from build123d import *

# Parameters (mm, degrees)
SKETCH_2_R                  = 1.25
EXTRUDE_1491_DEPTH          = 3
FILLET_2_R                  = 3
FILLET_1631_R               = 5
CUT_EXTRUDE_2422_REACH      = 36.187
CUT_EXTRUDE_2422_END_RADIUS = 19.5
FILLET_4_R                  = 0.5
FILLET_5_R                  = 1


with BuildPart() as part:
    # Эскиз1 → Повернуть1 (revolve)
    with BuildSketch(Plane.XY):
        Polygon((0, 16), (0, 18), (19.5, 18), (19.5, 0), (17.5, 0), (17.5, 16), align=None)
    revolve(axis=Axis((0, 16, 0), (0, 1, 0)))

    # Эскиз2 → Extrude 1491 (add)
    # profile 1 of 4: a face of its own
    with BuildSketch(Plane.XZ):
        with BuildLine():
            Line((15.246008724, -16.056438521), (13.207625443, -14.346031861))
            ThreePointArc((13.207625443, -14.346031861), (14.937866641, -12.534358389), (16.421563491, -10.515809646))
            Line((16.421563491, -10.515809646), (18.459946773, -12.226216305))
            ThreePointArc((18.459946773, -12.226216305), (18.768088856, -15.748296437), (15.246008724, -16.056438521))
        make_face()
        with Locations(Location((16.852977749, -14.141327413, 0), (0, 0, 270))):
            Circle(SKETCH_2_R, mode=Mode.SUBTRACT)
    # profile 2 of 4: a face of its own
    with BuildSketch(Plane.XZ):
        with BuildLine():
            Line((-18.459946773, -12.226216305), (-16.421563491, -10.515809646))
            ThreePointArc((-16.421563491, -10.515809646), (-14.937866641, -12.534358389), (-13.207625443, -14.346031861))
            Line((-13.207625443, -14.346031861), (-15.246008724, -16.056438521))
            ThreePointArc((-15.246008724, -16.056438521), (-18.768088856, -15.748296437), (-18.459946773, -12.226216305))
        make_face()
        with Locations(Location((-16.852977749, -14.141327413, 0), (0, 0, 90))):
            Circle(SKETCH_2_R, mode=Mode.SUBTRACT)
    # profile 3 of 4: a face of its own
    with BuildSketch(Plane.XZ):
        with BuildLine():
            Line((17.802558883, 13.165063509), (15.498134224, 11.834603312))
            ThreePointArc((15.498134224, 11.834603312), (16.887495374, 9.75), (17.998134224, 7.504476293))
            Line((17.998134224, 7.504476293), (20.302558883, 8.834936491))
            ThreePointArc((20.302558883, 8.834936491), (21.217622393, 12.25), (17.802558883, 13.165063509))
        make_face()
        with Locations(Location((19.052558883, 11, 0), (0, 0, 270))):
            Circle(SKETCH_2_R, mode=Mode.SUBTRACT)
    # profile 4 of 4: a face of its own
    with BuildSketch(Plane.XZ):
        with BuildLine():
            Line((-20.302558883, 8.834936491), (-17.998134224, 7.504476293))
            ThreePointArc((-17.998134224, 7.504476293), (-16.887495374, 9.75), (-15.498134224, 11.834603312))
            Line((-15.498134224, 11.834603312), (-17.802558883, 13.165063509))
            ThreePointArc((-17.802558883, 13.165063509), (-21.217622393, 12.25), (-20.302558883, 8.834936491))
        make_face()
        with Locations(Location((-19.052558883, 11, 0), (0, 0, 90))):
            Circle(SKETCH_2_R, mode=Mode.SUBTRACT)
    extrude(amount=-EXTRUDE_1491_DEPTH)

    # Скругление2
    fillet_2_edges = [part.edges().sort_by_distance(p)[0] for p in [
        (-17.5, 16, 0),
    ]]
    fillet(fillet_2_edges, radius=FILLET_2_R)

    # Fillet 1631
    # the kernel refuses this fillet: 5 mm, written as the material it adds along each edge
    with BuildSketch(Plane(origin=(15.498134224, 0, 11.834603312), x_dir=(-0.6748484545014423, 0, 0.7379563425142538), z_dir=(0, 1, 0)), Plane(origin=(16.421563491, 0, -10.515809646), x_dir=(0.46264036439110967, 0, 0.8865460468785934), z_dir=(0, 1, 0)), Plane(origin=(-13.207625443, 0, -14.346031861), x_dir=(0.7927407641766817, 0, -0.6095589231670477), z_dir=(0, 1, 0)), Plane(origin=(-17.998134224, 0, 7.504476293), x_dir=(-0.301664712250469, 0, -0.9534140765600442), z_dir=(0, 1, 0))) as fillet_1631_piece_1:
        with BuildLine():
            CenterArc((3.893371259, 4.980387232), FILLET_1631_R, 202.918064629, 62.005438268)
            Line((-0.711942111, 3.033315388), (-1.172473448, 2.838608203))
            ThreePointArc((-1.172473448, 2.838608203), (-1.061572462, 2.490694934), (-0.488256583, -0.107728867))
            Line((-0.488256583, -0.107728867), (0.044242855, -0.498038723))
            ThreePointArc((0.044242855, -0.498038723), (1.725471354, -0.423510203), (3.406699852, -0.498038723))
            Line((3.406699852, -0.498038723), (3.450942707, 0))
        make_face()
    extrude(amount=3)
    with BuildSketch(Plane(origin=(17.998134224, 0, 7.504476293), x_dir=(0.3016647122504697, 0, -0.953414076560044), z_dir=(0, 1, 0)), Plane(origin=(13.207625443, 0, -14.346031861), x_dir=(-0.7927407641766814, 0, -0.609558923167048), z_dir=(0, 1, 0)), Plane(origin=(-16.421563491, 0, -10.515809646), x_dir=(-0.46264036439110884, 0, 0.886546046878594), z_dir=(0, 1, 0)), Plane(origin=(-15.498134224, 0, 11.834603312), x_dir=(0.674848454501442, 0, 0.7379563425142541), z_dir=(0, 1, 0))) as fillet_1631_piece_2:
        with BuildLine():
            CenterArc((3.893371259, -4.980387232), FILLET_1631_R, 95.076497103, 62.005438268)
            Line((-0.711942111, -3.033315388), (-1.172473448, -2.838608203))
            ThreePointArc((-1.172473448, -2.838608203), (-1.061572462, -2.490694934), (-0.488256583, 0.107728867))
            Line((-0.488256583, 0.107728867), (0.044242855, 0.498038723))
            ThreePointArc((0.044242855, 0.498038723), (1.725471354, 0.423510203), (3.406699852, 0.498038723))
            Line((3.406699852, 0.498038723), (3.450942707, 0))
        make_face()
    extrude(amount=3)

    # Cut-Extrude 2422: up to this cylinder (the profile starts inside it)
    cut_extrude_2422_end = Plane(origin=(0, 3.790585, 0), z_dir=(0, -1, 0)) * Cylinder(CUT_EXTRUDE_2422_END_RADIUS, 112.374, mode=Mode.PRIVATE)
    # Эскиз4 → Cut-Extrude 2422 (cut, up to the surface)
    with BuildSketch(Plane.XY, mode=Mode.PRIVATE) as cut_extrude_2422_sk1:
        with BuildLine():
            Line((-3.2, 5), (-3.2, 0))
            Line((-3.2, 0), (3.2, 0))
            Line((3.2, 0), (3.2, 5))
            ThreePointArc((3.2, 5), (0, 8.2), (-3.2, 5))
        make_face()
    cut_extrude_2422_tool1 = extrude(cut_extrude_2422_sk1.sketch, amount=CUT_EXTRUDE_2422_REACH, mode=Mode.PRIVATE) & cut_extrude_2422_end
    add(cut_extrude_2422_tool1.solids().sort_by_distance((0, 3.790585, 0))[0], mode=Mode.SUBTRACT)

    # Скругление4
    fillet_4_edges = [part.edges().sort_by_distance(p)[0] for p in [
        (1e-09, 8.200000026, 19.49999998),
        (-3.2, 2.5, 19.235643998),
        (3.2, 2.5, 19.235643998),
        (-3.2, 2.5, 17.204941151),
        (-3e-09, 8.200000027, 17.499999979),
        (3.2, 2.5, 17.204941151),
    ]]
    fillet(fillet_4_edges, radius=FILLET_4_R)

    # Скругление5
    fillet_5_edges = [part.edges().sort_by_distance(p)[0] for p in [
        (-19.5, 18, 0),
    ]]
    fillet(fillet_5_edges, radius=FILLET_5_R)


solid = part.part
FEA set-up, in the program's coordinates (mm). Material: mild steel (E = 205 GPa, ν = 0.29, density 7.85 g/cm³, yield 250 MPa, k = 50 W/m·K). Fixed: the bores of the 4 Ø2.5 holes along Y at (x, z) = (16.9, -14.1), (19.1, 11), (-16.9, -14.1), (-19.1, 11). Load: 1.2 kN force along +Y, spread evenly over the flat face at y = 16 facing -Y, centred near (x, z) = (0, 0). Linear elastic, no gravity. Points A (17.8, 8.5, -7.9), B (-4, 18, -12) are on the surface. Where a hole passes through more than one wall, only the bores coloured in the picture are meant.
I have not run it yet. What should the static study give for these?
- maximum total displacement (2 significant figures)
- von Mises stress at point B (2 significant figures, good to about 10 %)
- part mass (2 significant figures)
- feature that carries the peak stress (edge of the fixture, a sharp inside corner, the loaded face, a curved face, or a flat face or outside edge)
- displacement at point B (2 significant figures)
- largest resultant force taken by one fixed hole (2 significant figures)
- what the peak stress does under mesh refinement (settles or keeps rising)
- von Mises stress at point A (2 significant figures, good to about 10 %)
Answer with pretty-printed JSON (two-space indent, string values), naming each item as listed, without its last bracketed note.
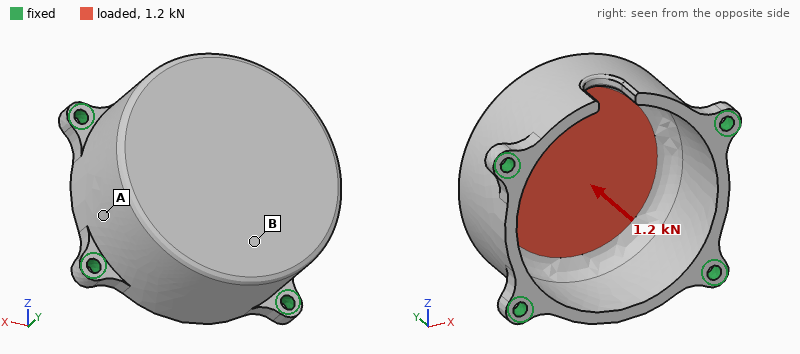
{
  "maximum total displacement": "23 µm",
  "von Mises stress at point B": "36 MPa",
  "part mass": "51 g",
  "feature that carries the peak stress": "edge of the fixture",
  "displacement at point B": "7.9 µm",
  "largest resultant force taken by one fixed hole": "350 N",
  "what the peak stress does under mesh refinement": "keeps rising",
  "von Mises stress at point A": "10 MPa"
}
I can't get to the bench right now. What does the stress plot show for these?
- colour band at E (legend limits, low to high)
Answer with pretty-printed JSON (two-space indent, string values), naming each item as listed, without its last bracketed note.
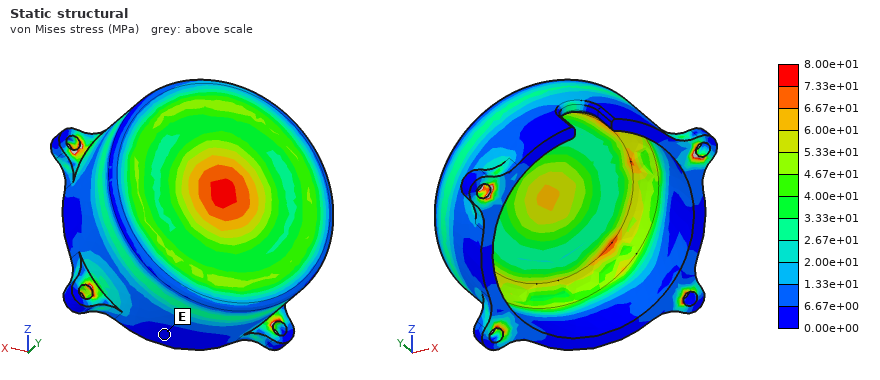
{
  "colour band at E": "0.00e+00 to 6.67e+00 MPa"
}
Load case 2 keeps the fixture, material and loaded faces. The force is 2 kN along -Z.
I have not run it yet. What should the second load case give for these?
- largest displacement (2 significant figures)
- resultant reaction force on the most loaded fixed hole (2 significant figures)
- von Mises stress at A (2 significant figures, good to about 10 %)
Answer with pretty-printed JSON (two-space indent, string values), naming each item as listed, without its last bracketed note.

{
  "largest displacement": "14 µm",
  "resultant reaction force on the most loaded fixed hole": "800 N",
  "von Mises stress at A": "34 MPa"
}
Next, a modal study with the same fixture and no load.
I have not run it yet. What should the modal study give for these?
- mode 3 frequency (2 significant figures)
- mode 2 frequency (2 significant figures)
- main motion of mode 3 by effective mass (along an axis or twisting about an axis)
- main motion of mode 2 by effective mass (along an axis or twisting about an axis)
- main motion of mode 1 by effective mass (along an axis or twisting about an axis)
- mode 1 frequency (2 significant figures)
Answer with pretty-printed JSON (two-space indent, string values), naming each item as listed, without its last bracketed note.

{
  "mode 3 frequency": "13 kHz",
  "mode 2 frequency": "13 kHz",
  "main motion of mode 3 by effective mass": "along Y",
  "main motion of mode 2 by effective mass": "along X",
  "main motion of mode 1 by effective mass": "along Z",
  "mode 1 frequency": "11 kHz"
}
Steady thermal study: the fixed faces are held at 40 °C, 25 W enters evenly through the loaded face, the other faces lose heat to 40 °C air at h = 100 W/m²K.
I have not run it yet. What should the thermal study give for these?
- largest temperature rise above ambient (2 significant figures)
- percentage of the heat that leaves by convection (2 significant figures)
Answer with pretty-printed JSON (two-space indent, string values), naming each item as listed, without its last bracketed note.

{
  "largest temperature rise above ambient": "55 K",
  "percentage of the heat that leaves by convection": "55 %"
}
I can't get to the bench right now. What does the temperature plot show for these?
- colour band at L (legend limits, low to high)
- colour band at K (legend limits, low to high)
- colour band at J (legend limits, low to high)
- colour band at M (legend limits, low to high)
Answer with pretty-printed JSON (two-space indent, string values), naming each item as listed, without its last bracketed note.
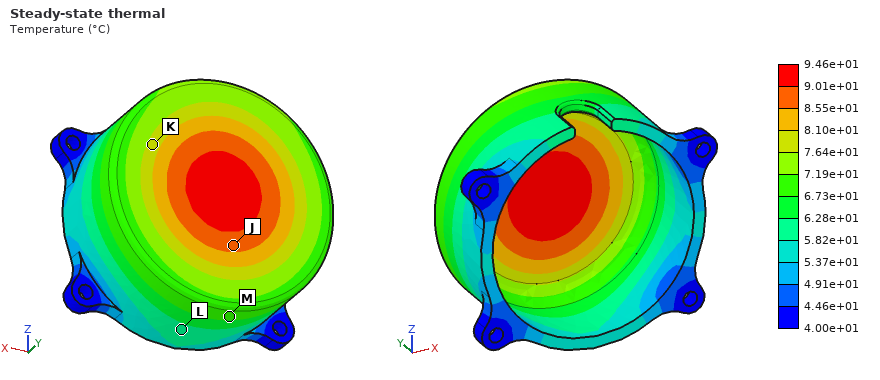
{
  "colour band at L": "5.82e+01 to 6.28e+01 °C",
  "colour band at K": "7.64e+01 to 8.10e+01 °C",
  "colour band at J": "8.55e+01 to 9.01e+01 °C",
  "colour band at M": "6.73e+01 to 7.19e+01 °C"
}
